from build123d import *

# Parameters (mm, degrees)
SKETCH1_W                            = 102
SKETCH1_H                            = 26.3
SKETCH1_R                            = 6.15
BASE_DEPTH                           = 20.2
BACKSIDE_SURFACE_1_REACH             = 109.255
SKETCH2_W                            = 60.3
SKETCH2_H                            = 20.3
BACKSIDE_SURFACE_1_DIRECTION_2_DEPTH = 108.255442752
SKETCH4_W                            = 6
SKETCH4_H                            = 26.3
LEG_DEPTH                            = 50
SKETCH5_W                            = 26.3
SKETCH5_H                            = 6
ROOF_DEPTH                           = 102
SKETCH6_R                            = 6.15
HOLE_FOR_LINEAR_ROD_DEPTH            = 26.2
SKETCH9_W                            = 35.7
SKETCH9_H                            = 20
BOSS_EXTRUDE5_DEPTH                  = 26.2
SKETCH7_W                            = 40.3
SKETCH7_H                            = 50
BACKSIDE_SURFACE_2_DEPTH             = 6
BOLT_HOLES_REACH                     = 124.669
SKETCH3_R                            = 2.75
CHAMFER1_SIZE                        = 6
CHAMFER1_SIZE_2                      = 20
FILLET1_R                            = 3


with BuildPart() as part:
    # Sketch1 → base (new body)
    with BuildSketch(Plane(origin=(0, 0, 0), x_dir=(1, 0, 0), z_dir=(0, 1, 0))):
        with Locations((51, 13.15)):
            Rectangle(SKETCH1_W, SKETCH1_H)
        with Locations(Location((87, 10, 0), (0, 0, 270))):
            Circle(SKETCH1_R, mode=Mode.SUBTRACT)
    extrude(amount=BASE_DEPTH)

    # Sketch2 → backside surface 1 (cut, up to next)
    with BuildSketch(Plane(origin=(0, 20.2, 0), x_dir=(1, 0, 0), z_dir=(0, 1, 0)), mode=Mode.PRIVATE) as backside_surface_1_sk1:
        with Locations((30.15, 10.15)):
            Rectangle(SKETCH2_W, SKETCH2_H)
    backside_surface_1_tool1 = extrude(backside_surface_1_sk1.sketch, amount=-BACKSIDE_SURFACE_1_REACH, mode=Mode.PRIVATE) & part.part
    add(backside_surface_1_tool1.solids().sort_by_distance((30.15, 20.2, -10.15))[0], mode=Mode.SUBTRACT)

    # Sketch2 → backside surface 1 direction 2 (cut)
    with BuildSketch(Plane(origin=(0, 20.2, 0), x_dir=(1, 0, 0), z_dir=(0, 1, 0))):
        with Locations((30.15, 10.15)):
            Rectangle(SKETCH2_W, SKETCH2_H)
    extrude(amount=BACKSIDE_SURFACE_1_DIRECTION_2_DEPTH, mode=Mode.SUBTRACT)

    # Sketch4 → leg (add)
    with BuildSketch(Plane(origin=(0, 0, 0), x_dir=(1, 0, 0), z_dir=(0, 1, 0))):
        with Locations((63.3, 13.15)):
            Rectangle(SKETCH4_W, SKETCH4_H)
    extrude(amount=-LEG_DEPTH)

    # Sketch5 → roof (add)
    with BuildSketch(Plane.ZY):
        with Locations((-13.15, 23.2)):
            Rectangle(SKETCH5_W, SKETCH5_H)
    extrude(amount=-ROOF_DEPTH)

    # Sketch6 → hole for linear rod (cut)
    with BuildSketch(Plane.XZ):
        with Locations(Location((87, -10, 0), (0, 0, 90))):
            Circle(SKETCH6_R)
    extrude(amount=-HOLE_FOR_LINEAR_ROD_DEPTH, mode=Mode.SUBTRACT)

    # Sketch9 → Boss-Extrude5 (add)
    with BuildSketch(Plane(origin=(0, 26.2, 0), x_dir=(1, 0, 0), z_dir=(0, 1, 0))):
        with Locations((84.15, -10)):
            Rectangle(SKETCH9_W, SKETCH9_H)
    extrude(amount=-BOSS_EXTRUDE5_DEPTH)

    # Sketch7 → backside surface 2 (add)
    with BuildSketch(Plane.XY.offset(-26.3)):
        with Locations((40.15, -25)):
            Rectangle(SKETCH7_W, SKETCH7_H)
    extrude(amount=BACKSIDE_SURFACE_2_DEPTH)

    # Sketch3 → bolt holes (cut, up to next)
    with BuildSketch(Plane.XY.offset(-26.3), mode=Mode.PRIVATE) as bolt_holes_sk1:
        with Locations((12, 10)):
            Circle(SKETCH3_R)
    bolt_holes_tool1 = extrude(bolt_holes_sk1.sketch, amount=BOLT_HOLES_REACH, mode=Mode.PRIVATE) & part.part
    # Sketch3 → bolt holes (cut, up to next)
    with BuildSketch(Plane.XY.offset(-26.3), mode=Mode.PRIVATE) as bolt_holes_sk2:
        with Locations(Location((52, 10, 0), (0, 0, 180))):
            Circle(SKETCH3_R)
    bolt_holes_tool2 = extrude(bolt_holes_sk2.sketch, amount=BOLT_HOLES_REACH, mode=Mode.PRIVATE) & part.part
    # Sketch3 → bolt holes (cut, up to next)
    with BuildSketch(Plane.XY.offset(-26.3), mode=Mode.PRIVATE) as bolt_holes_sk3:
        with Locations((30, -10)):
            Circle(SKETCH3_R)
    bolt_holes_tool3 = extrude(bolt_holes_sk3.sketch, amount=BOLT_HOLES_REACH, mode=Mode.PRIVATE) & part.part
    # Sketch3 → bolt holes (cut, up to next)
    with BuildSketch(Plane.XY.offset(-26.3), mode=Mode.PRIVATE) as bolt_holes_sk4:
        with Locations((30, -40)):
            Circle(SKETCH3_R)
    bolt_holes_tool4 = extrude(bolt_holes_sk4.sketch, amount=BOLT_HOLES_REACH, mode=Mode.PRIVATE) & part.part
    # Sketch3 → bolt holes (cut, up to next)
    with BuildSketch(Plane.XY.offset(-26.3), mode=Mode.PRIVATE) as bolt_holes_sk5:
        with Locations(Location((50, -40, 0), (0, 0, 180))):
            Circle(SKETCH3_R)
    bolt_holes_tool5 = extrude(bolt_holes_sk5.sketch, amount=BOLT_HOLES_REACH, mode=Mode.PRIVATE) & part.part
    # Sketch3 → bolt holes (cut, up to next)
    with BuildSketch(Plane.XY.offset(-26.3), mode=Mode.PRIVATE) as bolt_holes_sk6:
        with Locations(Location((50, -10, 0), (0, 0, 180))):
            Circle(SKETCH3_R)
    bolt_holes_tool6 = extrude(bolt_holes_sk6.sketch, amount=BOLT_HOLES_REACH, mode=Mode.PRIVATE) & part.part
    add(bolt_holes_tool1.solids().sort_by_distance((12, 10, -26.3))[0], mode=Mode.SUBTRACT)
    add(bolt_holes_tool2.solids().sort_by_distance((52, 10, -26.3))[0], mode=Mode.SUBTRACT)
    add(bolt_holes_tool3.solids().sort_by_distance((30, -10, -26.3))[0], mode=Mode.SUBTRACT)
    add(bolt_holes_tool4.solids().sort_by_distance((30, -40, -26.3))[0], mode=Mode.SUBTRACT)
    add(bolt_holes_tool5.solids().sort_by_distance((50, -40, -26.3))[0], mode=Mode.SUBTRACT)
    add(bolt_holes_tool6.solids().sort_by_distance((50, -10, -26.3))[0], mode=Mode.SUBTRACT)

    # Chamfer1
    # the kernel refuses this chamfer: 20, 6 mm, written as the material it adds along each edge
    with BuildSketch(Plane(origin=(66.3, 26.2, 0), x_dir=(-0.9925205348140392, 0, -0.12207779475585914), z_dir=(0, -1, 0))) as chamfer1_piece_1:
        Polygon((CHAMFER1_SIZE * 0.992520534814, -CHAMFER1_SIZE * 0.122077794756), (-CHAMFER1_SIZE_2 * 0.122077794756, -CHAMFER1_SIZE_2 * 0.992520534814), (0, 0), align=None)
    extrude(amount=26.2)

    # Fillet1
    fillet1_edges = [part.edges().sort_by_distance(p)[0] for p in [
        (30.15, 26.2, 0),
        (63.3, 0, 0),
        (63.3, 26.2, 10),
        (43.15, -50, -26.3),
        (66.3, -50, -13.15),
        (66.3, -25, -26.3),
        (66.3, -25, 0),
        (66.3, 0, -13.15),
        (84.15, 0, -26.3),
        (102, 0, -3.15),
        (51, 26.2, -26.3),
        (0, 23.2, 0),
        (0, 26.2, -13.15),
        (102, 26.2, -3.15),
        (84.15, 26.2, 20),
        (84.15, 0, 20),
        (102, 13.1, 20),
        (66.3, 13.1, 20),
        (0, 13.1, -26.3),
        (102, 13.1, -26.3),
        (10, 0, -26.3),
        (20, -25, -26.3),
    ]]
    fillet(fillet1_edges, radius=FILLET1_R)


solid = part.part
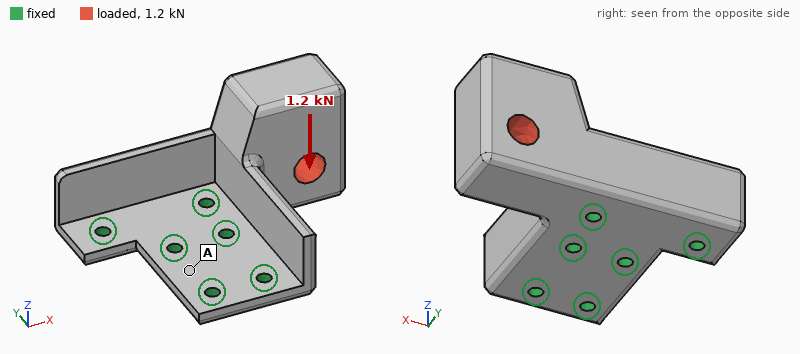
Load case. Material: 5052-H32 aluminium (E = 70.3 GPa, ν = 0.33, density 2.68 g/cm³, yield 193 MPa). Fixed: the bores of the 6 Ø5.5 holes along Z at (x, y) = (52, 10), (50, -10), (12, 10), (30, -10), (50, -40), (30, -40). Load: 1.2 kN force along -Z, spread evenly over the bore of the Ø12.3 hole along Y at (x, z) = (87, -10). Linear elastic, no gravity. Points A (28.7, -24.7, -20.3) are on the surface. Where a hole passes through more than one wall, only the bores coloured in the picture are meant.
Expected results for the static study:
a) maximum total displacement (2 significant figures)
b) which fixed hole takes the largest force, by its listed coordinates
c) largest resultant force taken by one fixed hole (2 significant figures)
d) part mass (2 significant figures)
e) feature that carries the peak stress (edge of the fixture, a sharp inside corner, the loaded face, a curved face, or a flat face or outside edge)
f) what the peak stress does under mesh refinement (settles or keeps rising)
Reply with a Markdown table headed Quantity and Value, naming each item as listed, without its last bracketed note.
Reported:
| Quantity | Value |
|---|---|
| maximum total displacement | 0.11 mm |
| which fixed hole takes the largest force, by its listed coordinates | (52, 10) |
| largest resultant force taken by one fixed hole | 2.1 kN |
| part mass | 220 g |
| feature that carries the peak stress | edge of the fixture |
| what the peak stress does under mesh refinement | keeps rising |
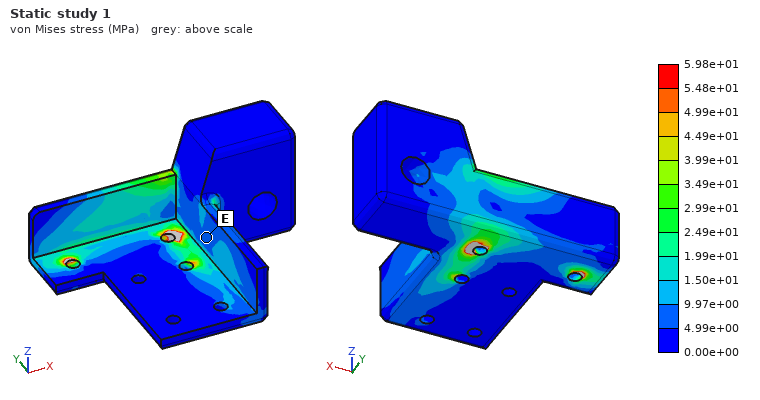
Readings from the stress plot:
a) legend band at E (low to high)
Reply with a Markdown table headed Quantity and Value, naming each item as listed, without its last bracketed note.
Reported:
| Quantity | Value |
|---|---|
| legend band at E | 4.99e+00 to 9.97e+00 MPa |
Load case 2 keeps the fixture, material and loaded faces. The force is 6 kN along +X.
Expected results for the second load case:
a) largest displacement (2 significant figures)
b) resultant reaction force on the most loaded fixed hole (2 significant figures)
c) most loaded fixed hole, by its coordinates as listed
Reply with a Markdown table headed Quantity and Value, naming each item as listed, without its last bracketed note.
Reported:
| Quantity | Value |
|---|---|
| largest displacement | 0.18 mm |
| resultant reaction force on the most loaded fixed hole | 3.6 kN |
| most loaded fixed hole, by its coordinates as listed | (52, 10) |
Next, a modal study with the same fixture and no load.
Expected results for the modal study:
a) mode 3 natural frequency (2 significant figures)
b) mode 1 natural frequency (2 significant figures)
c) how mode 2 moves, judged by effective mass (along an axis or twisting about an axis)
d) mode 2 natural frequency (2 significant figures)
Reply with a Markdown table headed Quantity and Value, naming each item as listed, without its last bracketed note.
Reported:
| Quantity | Value |
|---|---|
| mode 3 natural frequency | 5400 Hz |
| mode 1 natural frequency | 1800 Hz |
| how mode 2 moves, judged by effective mass | along Y |
| mode 2 natural frequency | 3700 Hz |
